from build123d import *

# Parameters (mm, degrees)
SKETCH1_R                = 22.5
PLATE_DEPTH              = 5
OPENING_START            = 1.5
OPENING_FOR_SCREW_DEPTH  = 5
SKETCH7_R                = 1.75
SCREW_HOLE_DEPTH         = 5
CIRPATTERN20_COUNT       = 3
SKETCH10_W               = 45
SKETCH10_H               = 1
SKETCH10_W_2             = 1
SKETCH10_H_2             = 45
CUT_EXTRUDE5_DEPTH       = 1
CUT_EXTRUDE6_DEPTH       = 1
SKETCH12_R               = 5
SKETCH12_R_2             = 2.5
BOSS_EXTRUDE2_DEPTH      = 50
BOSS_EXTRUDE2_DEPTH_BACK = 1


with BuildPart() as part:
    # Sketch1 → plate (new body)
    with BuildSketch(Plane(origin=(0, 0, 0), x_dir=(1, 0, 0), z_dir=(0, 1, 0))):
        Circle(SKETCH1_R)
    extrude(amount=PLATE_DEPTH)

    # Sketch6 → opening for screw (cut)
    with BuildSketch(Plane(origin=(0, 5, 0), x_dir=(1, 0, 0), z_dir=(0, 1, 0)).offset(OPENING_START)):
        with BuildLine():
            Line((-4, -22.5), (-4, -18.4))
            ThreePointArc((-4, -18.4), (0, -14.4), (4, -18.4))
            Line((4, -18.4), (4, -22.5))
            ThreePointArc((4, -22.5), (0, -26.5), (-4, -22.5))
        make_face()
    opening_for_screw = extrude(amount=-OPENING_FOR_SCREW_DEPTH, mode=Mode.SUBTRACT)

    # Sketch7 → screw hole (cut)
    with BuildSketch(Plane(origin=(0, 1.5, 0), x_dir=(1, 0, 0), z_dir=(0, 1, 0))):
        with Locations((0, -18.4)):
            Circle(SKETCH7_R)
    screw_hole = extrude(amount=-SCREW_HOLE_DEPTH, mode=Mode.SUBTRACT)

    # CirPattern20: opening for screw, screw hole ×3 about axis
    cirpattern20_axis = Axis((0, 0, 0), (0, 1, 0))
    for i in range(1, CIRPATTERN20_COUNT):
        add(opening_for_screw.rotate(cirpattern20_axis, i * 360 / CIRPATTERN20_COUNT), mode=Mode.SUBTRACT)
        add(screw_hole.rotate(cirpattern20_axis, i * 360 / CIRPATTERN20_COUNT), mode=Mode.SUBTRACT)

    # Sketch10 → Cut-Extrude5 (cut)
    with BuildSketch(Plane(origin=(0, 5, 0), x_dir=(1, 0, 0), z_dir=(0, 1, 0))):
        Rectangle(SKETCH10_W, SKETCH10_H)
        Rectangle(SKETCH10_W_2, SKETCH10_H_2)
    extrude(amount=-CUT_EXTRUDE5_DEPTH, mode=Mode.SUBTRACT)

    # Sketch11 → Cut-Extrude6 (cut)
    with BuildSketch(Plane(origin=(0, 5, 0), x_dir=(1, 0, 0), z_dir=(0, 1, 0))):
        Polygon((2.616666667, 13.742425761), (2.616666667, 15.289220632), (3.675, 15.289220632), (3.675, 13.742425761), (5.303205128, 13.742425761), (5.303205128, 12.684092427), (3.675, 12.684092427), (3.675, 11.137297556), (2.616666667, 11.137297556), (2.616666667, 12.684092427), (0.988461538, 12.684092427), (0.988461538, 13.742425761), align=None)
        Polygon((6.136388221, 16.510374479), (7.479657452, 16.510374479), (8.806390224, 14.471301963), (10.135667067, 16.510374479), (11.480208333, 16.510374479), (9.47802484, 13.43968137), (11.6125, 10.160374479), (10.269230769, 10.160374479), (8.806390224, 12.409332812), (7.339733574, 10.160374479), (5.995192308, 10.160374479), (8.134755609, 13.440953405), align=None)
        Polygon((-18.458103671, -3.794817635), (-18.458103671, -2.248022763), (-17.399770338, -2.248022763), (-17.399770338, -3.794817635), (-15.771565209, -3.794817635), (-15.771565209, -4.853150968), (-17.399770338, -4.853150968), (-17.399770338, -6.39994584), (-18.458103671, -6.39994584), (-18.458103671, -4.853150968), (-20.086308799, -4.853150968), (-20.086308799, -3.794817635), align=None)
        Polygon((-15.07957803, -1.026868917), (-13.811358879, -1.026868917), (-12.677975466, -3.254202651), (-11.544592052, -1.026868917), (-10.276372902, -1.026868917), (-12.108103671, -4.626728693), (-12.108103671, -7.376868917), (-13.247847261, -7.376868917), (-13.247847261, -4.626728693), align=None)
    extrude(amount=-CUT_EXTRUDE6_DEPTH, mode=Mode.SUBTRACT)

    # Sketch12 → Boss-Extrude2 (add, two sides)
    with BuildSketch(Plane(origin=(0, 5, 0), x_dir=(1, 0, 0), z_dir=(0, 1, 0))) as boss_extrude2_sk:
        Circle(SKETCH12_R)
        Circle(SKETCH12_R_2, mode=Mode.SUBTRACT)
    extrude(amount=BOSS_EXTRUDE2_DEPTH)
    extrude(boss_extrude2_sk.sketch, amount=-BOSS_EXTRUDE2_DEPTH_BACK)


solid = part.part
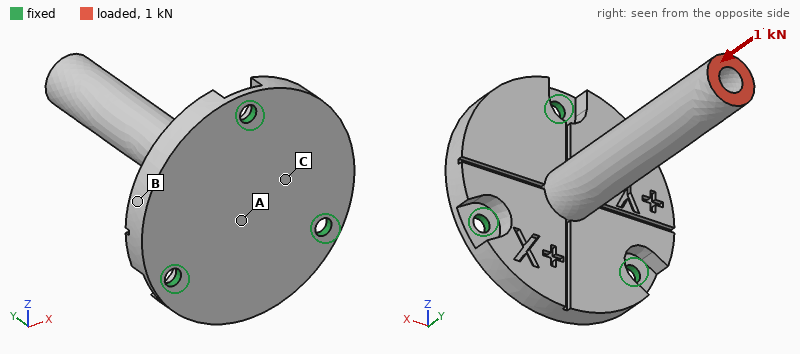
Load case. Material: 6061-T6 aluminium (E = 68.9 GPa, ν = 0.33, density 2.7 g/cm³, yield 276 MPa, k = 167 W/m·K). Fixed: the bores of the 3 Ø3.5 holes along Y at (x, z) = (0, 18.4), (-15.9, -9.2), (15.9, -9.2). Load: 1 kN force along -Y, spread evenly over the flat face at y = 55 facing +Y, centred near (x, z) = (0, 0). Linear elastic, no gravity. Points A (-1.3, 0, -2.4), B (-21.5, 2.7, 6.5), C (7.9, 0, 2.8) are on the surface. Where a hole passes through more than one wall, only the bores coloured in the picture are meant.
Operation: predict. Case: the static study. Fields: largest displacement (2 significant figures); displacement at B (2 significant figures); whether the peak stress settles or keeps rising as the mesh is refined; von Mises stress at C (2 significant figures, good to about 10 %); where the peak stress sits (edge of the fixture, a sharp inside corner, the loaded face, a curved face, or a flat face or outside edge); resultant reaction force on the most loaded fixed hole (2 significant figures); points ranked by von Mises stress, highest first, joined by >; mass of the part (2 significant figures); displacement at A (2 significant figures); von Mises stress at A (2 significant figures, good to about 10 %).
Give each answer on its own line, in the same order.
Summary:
31 µm
5.5 µm
keeps rising
20 MPa
edge of the fixture
480 N
A > C > B
27 g
19 µm
28 MPa
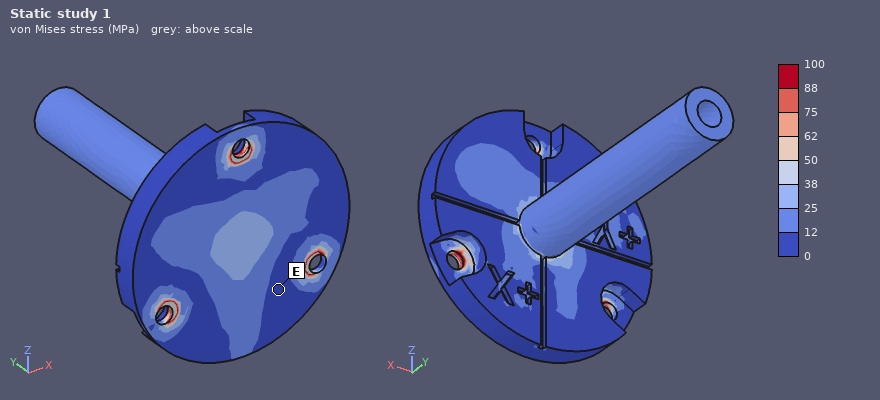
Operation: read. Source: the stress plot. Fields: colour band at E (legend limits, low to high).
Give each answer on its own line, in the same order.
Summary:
0 to 12 MPa
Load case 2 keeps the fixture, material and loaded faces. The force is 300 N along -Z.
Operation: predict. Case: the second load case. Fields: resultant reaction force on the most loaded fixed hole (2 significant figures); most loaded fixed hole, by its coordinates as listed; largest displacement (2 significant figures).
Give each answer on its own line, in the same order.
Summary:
780 N
(0, 18.4)
0.59 mm
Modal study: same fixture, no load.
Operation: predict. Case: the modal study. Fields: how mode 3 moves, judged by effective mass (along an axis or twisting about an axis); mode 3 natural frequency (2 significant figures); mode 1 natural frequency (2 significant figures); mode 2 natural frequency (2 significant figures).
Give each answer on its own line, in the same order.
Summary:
along Y
9200 Hz
2400 Hz
2400 Hz
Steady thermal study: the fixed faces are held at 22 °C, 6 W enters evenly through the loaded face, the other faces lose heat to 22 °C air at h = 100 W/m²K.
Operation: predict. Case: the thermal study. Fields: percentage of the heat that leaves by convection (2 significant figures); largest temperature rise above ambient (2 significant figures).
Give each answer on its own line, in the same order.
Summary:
52 %
24 K
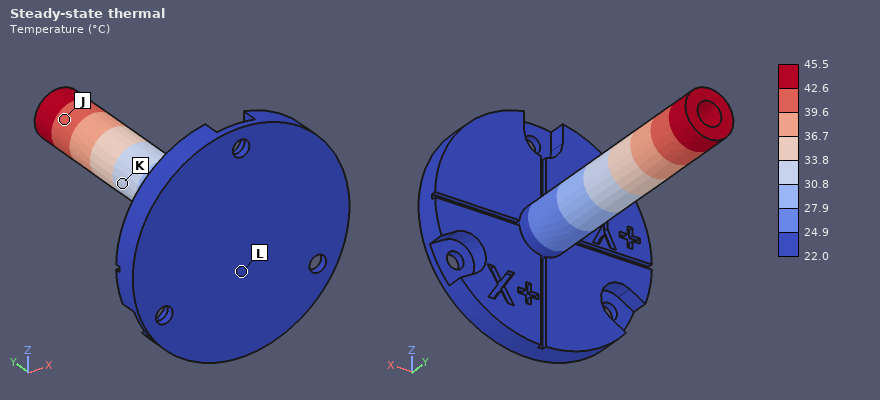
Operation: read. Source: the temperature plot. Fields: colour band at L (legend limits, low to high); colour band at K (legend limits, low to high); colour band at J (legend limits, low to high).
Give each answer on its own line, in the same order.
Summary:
22.0 to 24.9 °C
30.8 to 33.8 °C
39.6 to 42.6 °C
